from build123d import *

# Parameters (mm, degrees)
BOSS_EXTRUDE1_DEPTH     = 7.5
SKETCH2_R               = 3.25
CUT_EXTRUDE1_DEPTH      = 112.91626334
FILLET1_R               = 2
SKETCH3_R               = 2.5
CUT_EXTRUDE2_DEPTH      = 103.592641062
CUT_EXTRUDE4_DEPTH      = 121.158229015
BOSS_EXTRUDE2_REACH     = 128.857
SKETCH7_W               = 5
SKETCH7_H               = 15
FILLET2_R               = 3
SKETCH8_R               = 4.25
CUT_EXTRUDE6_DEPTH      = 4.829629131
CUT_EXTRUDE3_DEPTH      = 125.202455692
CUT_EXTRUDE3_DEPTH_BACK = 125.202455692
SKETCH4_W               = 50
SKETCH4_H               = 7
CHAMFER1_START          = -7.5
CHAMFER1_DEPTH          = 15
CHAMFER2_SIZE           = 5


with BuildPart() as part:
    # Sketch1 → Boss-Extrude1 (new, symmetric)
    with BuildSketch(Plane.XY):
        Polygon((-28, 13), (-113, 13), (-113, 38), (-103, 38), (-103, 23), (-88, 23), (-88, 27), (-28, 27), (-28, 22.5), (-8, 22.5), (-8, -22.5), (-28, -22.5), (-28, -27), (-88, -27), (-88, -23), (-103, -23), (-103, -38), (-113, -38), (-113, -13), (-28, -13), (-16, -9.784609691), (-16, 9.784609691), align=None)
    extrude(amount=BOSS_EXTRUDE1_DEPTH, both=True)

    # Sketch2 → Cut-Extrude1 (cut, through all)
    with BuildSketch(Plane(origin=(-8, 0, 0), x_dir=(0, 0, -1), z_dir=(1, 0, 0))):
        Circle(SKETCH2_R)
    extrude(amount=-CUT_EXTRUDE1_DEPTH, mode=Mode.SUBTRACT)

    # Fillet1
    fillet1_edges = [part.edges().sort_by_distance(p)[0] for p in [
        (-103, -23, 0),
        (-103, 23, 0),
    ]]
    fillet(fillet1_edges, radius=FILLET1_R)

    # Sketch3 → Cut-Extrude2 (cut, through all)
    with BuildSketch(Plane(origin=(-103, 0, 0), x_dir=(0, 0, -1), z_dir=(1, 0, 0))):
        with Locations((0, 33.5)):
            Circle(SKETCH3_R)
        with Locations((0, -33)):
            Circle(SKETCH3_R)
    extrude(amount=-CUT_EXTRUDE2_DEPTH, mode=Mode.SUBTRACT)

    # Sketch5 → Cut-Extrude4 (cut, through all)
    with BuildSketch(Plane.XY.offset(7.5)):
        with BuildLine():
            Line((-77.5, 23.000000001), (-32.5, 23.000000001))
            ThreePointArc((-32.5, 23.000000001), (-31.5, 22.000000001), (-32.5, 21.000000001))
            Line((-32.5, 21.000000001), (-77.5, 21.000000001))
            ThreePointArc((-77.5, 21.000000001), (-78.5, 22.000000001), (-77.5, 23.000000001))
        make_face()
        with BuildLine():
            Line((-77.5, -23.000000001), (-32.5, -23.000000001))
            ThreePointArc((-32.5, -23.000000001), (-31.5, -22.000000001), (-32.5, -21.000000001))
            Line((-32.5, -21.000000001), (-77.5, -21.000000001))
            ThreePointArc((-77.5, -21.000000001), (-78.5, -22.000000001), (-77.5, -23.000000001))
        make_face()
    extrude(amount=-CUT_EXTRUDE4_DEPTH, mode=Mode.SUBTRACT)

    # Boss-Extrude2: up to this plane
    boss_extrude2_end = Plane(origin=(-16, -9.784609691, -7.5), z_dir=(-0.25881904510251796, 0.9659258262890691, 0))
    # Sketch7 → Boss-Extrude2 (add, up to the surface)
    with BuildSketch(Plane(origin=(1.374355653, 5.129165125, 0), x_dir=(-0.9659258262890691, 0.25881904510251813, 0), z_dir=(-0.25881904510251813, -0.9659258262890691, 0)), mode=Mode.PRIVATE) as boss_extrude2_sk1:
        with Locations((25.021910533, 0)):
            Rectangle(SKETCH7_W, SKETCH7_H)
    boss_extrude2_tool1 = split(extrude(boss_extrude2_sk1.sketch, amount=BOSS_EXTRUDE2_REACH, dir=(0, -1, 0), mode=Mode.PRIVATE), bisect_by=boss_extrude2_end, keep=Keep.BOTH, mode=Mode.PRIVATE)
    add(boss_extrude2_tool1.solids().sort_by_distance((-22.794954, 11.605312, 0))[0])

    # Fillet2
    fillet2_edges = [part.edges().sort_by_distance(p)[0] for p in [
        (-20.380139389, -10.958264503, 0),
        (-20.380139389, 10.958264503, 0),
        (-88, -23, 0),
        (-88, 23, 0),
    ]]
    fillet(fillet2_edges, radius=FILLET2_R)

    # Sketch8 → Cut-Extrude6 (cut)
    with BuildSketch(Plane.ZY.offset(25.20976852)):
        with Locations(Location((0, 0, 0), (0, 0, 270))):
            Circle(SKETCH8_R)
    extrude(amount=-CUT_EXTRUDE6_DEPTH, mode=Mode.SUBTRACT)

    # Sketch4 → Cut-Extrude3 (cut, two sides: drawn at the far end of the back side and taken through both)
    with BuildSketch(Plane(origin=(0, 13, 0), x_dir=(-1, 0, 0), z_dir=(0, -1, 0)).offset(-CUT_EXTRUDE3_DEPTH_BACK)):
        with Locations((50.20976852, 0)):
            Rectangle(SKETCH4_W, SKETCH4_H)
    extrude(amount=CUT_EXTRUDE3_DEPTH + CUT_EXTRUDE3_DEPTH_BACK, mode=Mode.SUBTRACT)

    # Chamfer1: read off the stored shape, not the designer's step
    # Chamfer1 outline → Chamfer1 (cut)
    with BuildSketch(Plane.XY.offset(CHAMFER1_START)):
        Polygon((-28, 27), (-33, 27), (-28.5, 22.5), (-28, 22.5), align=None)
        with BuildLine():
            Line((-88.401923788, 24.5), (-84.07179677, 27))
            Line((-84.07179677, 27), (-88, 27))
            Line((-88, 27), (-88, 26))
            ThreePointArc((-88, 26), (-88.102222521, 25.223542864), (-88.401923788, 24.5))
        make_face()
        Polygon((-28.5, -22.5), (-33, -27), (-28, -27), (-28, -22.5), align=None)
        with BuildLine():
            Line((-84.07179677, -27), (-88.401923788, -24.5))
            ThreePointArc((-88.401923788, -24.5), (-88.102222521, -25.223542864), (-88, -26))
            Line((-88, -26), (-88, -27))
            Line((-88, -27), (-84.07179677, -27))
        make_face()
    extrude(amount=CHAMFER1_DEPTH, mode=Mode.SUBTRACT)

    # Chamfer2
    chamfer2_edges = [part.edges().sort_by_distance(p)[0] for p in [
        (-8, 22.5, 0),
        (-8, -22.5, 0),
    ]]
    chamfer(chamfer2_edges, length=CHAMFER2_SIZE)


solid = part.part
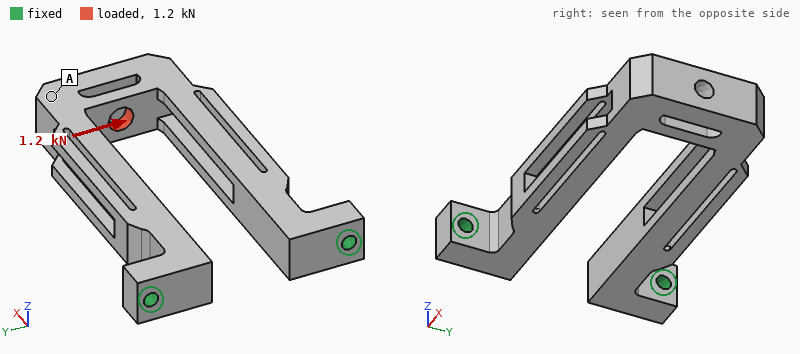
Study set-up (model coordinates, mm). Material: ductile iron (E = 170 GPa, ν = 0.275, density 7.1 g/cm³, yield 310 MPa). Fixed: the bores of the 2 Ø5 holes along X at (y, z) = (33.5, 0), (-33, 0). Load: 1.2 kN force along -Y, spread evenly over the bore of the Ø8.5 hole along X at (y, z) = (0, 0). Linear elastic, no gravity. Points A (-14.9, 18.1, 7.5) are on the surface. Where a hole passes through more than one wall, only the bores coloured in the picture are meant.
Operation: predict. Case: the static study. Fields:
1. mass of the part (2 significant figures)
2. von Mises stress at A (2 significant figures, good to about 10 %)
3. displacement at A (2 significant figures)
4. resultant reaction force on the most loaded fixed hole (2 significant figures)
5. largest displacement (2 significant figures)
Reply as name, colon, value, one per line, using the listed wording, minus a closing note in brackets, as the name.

mass of the part: 250 g
von Mises stress at A: 22 MPa
displacement at A: 0.30 mm
resultant reaction force on the most loaded fixed hole: 1.4 kN
largest displacement: 0.30 mm
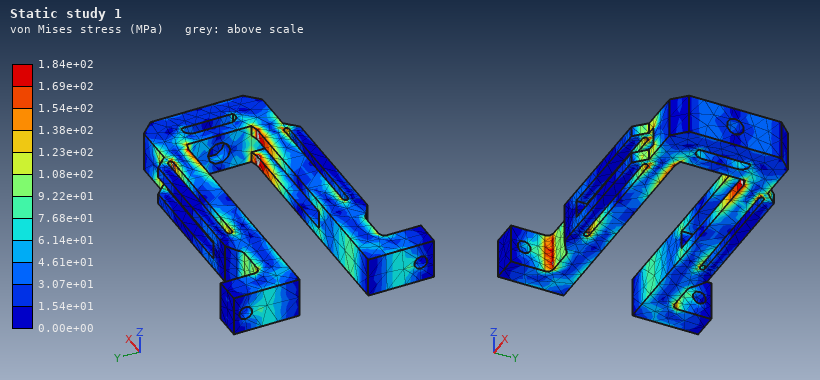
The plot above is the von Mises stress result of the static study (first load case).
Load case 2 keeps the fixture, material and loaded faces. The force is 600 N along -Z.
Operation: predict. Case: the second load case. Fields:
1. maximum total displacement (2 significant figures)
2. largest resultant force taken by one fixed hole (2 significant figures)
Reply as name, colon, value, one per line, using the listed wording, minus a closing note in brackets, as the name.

maximum total displacement: 0.48 mm
largest resultant force taken by one fixed hole: 300 N
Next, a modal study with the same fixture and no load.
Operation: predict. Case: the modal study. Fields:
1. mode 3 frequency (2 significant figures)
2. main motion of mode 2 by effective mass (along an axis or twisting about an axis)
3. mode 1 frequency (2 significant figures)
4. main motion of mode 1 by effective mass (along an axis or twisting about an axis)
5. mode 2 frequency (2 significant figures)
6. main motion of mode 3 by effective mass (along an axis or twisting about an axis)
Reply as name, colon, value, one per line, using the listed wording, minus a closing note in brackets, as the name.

mode 3 frequency: 1400 Hz
main motion of mode 2 by effective mass: along Y
mode 1 frequency: 590 Hz
main motion of mode 1 by effective mass: along Z
mode 2 frequency: 990 Hz
main motion of mode 3 by effective mass: twisting about X
